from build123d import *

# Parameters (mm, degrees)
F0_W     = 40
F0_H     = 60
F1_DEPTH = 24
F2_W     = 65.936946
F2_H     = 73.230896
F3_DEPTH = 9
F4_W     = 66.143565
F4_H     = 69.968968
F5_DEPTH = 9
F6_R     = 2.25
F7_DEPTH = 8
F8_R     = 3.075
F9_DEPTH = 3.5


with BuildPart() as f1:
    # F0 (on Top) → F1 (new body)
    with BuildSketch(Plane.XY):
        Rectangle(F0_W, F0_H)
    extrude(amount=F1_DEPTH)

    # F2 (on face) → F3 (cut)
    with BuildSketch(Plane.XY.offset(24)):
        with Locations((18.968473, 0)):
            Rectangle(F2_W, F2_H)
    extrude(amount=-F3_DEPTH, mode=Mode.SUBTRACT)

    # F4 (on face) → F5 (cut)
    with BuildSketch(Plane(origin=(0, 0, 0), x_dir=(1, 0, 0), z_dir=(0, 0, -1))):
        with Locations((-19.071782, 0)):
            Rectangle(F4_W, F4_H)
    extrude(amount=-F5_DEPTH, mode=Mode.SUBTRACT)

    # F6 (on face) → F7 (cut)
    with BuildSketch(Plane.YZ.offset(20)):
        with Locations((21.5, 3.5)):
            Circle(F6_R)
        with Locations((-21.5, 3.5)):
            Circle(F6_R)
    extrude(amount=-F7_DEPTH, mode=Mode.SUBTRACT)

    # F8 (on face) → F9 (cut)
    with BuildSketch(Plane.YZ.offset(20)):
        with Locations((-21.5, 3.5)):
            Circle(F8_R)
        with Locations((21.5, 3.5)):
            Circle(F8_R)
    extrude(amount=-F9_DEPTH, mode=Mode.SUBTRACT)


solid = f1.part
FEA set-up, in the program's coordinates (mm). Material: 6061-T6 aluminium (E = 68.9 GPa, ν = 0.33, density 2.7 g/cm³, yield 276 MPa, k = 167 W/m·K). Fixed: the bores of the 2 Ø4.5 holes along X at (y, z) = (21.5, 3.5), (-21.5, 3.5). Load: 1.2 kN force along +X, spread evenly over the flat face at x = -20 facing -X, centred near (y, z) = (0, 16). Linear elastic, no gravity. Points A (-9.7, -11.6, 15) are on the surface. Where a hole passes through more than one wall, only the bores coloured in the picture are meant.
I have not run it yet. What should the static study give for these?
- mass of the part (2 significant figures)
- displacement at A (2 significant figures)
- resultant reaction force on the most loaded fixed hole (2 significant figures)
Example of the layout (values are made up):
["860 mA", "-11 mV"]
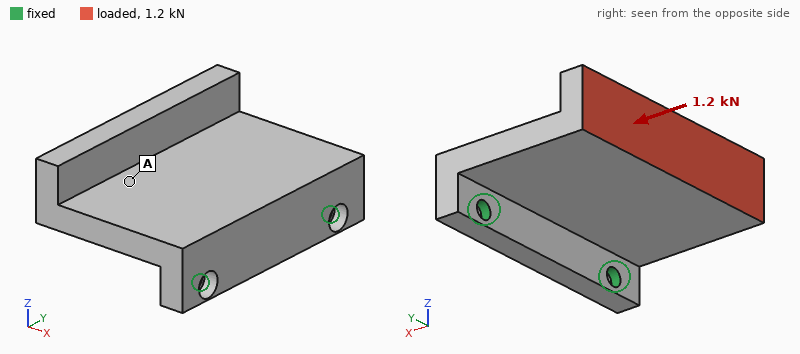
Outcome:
["56 g", "0.17 mm", "600 N"]
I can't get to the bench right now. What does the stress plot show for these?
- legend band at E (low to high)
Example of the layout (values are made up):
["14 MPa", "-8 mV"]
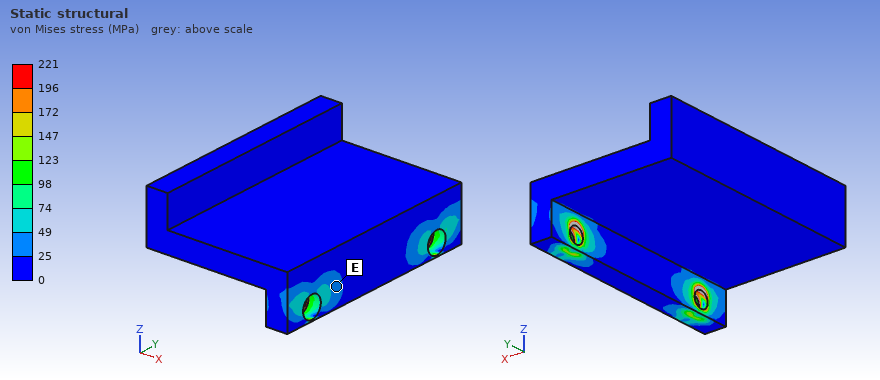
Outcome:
["25 to 49 MPa"]
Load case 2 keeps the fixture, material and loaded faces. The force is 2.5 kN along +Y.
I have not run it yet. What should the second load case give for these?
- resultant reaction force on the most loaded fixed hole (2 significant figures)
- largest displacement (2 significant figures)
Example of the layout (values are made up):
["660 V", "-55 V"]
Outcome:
["2.5 kN", "88 µm"]
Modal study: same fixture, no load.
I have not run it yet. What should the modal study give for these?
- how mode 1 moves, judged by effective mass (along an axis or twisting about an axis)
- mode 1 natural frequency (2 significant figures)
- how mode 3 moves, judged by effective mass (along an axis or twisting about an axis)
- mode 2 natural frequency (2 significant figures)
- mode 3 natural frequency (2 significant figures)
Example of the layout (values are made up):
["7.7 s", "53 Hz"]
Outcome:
["along Z", "1300 Hz", "along Y", "4000 Hz", "5900 Hz"]
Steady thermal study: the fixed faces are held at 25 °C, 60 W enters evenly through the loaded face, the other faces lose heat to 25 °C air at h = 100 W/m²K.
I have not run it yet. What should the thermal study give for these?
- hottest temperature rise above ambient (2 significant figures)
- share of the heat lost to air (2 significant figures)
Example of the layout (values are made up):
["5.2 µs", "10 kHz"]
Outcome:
["43 K", "30 %"]
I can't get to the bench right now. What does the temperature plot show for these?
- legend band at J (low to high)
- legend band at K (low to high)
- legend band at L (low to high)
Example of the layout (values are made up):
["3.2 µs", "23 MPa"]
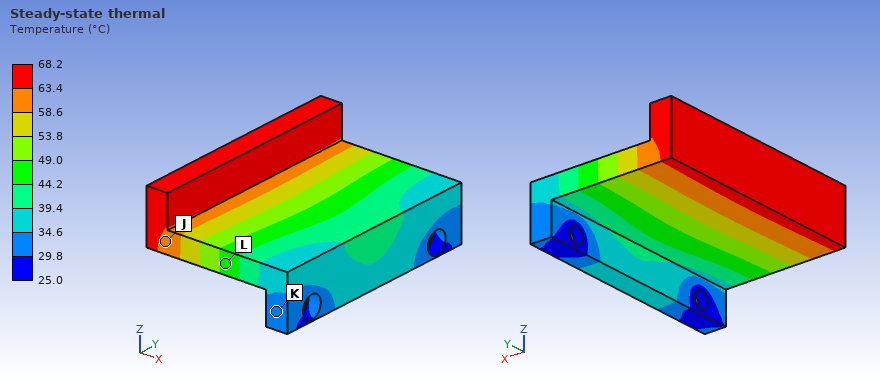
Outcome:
["58.6 to 63.4 °C", "29.8 to 34.6 °C", "44.2 to 49.0 °C"]
